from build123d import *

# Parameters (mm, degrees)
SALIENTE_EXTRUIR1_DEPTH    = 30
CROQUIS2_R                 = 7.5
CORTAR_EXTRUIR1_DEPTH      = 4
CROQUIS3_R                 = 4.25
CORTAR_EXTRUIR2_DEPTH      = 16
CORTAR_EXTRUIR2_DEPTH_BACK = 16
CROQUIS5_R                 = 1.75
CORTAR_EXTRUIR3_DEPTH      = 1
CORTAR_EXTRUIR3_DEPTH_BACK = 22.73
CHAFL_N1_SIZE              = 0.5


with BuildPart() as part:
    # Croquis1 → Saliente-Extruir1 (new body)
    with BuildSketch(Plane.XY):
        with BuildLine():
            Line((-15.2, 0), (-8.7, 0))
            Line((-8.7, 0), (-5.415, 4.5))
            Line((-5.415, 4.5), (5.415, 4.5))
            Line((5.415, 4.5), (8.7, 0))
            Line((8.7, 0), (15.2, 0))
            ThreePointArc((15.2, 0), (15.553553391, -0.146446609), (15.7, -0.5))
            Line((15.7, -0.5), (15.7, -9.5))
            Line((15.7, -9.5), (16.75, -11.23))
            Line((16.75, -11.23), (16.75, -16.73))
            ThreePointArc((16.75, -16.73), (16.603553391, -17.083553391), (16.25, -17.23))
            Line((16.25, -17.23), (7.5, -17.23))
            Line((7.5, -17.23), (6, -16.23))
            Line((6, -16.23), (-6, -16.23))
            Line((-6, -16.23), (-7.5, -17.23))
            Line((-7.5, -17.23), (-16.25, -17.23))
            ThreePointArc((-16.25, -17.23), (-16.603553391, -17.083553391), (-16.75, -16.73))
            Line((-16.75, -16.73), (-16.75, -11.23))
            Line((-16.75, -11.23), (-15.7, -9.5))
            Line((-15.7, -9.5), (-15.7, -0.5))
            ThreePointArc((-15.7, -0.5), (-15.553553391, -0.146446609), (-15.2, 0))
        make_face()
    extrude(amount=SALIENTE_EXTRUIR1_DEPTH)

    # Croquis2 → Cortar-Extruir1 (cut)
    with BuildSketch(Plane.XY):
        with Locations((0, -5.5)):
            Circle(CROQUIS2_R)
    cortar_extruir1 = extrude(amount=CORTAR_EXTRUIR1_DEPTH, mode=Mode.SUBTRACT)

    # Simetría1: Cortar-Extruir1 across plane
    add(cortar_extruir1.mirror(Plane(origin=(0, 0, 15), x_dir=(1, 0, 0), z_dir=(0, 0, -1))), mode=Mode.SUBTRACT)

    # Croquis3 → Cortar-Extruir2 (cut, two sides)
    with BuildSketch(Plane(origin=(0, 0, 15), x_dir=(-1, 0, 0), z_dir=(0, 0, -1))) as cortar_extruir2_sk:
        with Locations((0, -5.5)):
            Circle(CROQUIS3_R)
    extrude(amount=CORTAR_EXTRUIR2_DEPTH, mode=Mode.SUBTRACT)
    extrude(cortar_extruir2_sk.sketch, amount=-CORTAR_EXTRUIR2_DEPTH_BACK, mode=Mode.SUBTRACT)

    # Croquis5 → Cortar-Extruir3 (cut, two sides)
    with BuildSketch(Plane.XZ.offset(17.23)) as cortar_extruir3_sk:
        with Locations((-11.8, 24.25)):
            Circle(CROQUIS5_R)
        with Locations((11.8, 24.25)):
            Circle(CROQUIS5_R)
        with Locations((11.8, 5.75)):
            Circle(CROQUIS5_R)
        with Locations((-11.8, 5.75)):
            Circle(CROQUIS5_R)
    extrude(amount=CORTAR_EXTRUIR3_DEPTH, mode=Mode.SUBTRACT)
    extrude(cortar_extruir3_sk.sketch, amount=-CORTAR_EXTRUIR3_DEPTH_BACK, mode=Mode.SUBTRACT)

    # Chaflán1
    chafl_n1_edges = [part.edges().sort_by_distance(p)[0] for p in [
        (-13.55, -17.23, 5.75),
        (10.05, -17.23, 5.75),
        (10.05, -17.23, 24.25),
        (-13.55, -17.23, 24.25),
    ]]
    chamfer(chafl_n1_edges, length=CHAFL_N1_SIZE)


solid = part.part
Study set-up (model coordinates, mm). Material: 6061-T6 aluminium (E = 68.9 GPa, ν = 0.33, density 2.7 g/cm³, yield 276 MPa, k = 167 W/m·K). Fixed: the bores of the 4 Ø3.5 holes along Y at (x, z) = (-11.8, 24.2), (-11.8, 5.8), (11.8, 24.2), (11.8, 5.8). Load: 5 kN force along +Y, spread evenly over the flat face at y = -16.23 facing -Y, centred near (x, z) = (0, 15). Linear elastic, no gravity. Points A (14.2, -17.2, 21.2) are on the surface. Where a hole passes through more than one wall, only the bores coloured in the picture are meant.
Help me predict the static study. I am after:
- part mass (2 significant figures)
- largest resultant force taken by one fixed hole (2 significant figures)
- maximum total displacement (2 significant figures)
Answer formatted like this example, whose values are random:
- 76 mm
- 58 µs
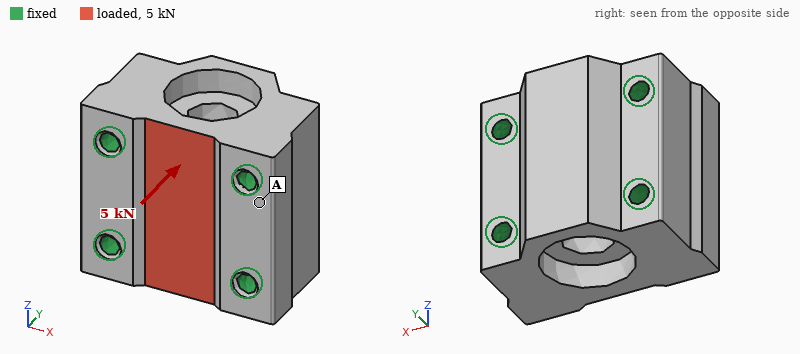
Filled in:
- 40 g
- 1.3 kN
- 7.1 µm
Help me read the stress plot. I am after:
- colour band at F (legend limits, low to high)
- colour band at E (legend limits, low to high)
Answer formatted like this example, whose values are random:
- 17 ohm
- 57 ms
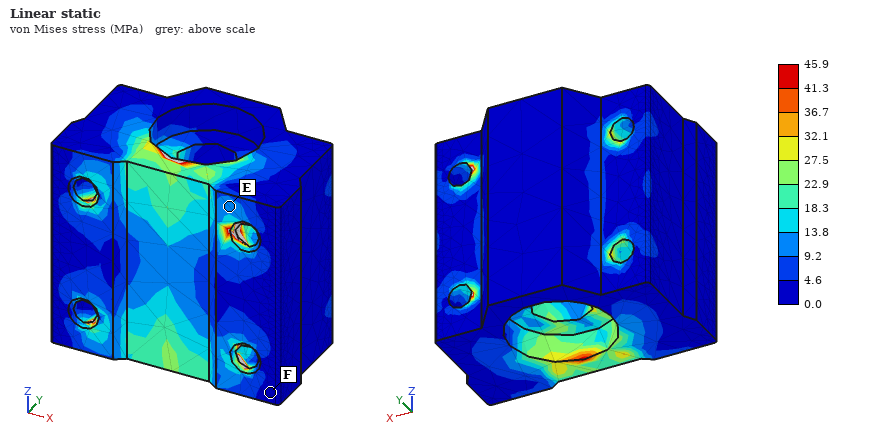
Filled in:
- 0.0 to 4.6 MPa
- 9.2 to 13.8 MPa
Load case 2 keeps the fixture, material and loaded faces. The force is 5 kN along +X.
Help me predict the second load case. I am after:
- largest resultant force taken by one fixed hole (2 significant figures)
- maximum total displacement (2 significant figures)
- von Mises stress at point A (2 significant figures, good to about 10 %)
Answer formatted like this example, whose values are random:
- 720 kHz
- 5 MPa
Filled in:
- 1.4 kN
- 2.9 µm
- 8.4 MPa
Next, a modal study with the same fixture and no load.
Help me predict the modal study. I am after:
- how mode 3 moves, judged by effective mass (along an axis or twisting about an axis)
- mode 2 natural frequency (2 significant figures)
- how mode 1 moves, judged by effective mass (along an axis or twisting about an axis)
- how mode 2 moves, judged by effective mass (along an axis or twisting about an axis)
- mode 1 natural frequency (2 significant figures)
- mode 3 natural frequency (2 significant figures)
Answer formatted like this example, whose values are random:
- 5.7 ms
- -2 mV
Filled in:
- along X
- 55 kHz
- along Z
- along Y
- 52 kHz
- 66 kHz
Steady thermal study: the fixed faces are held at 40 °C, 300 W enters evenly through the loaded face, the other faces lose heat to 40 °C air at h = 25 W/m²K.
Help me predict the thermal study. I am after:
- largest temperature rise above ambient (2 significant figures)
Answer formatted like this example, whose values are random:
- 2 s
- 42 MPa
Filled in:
- 44 K
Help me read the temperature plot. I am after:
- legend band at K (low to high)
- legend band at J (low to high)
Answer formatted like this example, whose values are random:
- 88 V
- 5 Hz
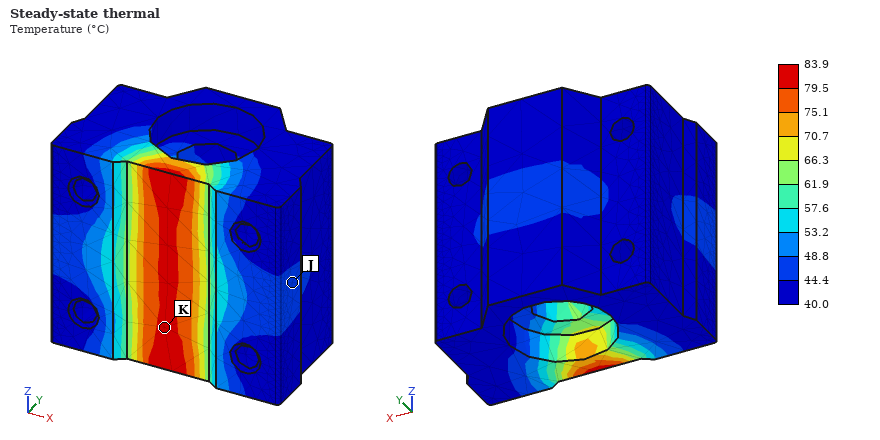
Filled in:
- 79.5 to 83.9 °C
- 44.4 to 48.8 °C
